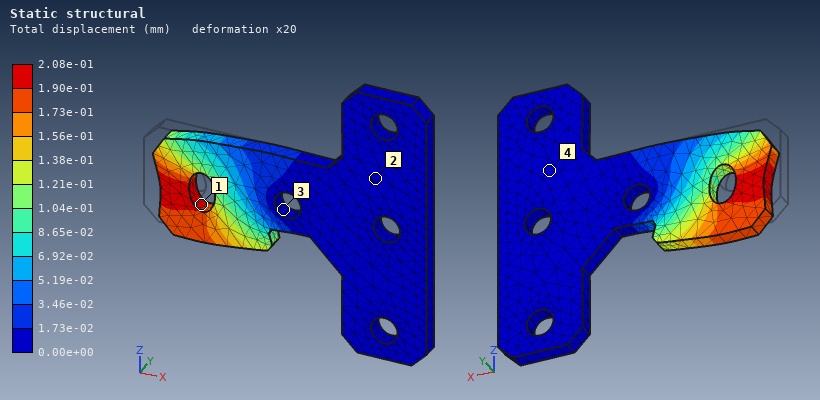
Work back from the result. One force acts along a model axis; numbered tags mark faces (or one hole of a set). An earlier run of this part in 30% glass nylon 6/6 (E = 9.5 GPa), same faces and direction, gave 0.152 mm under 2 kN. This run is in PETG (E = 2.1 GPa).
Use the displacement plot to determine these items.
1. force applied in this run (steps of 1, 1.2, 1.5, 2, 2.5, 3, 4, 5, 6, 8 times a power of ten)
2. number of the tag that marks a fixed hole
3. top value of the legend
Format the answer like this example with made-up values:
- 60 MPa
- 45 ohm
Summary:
- 600 N
- 3
- 2.08e-01 mm
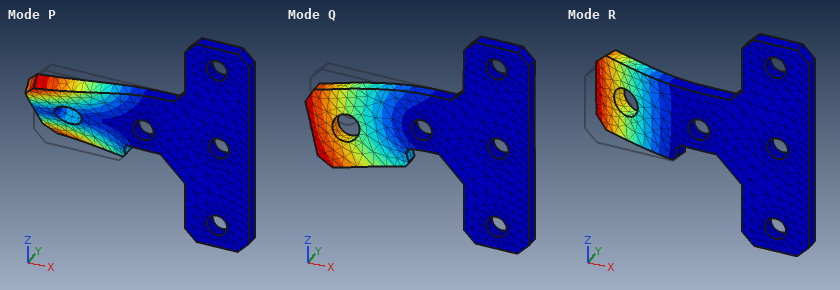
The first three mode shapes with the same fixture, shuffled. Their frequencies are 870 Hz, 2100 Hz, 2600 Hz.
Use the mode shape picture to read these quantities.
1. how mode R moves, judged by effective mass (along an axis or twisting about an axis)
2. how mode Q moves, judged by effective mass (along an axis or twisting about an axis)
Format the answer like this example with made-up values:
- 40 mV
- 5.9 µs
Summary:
- along Y
- along Z
